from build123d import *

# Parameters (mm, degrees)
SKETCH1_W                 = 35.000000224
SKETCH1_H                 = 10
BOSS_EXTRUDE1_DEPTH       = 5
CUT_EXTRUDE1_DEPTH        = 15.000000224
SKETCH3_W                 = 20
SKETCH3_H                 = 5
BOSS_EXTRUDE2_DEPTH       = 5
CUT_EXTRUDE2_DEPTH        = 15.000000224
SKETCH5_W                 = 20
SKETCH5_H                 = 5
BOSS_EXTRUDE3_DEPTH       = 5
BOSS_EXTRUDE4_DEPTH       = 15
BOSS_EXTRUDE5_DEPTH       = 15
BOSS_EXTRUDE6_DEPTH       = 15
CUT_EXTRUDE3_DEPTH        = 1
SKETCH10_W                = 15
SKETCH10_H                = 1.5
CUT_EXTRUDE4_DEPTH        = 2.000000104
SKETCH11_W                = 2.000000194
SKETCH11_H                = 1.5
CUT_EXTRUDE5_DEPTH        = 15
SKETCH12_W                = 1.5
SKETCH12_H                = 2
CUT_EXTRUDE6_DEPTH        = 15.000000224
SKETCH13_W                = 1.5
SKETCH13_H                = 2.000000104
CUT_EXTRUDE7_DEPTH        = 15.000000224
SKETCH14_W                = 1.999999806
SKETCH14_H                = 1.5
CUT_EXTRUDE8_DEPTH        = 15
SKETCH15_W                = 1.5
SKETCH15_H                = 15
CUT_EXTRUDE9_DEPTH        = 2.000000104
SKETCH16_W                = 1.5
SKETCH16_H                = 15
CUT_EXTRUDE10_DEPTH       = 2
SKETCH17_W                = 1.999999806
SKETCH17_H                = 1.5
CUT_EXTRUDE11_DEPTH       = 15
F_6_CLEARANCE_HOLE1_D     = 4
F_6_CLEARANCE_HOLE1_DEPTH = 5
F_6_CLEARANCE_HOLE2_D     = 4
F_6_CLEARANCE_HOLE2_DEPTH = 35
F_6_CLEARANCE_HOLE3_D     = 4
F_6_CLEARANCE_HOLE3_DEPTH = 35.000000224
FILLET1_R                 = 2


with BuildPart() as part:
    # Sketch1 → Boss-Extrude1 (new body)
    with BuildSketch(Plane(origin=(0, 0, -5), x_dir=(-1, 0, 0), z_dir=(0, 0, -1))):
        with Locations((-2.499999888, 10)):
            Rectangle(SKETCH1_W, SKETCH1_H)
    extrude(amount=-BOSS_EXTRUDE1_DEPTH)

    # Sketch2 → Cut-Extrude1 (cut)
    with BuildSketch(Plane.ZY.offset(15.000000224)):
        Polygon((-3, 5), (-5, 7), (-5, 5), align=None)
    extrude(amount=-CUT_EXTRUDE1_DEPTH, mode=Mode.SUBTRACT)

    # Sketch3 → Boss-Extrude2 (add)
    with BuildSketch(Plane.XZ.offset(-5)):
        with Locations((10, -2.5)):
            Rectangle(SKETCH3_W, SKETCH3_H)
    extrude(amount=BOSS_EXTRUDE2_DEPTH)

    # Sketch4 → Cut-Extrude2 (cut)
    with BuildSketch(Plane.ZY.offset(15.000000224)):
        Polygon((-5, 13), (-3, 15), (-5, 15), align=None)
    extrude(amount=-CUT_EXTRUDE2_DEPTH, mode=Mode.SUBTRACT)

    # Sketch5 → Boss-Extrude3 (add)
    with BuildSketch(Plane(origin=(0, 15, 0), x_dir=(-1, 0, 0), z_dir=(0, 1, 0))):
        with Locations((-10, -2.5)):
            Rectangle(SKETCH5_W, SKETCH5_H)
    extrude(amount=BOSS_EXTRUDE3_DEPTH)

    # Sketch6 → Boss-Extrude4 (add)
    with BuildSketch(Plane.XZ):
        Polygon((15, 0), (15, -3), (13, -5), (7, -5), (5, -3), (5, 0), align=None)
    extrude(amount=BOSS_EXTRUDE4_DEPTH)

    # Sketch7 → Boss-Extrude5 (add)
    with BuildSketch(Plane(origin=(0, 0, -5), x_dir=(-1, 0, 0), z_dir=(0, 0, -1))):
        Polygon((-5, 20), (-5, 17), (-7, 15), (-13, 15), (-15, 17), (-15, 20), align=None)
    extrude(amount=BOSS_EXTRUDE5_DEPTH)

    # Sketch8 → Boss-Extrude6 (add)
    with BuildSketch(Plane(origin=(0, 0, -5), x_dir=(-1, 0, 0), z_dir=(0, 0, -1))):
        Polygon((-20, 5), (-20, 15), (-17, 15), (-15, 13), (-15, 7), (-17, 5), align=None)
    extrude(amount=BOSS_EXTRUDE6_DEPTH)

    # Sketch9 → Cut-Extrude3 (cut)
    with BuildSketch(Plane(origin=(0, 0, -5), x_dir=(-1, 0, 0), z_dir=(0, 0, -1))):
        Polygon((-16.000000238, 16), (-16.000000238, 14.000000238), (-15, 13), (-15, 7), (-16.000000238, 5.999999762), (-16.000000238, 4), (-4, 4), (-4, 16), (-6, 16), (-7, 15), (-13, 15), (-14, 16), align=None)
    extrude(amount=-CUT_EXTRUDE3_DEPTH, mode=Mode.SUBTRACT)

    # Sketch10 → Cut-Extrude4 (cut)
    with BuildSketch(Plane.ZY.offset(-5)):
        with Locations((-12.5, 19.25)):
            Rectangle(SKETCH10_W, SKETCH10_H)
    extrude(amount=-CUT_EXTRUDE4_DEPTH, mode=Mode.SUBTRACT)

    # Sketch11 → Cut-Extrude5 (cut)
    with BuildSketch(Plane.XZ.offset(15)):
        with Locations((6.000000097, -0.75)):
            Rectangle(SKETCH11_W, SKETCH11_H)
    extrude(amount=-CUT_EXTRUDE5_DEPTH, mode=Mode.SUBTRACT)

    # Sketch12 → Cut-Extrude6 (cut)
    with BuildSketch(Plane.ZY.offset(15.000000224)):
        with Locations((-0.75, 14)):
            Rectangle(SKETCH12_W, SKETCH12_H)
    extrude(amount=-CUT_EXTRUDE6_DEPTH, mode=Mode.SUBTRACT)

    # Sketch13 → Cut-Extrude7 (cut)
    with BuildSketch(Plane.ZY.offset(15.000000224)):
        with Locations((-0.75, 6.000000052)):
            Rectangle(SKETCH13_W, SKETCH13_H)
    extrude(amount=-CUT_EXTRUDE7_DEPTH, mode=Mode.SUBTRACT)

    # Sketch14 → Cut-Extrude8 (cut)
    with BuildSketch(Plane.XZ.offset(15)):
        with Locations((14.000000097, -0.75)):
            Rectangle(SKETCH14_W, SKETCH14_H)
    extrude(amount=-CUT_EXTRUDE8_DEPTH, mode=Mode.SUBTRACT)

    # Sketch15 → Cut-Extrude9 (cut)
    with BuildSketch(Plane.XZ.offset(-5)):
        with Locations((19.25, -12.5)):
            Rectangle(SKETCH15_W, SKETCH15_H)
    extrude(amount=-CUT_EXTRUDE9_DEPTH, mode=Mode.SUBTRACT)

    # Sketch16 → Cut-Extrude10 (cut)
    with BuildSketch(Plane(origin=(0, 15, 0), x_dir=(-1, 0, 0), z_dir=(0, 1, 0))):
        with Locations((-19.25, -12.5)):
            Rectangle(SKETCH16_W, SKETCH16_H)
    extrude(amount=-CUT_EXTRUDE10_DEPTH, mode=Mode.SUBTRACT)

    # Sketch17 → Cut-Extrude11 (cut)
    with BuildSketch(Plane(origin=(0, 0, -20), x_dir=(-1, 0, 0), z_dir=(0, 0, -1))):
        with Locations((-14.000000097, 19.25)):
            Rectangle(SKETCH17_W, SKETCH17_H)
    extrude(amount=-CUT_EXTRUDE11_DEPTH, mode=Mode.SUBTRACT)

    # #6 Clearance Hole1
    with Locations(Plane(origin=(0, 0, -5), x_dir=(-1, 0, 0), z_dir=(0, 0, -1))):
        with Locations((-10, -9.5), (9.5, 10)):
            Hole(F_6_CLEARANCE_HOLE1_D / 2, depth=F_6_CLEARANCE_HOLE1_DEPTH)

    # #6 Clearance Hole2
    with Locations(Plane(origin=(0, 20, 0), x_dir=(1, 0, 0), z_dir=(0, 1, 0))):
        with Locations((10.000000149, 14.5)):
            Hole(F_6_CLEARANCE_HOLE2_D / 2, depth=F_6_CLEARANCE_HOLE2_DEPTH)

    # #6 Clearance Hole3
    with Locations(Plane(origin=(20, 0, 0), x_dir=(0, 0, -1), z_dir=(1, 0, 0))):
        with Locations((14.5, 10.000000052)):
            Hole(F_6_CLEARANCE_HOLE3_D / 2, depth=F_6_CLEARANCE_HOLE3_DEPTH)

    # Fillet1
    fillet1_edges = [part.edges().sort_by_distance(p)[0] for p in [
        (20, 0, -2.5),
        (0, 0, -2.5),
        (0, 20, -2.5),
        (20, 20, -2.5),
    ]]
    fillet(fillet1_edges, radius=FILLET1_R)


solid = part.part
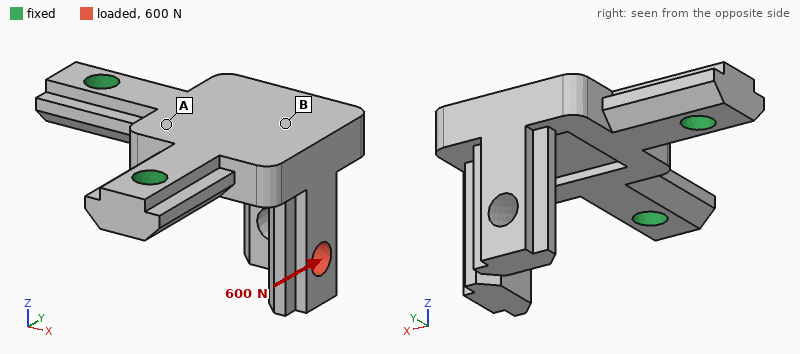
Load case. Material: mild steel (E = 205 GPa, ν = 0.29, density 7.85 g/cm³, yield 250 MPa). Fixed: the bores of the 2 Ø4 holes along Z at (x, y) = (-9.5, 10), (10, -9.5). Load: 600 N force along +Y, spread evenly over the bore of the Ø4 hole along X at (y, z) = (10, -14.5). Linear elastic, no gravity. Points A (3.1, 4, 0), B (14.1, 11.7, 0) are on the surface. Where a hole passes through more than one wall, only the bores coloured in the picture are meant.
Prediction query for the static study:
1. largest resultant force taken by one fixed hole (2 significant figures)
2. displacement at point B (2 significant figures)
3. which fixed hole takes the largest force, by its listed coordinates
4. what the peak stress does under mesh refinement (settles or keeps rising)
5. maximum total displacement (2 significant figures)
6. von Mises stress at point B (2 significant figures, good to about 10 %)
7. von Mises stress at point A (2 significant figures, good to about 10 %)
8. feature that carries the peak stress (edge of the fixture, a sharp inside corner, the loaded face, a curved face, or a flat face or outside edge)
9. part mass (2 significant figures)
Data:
710 N
33 µm
(10, -9.5)
keeps rising
96 µm
69 MPa
25 MPa
a sharp inside corner
31 g
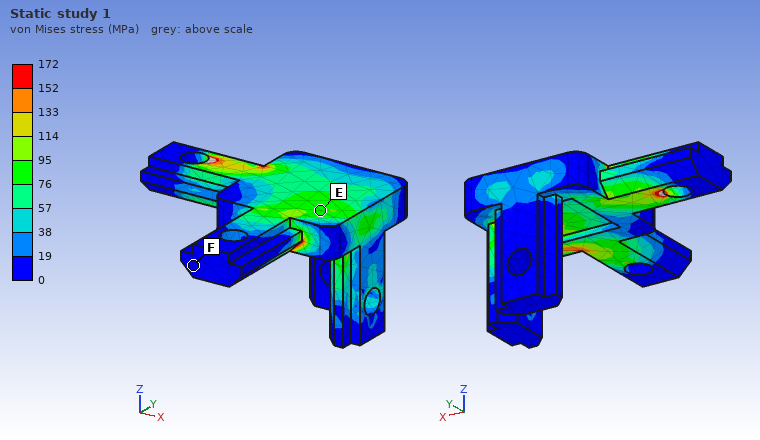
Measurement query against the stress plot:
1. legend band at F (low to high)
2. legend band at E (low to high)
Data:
0 to 19 MPa
76 to 95 MPa
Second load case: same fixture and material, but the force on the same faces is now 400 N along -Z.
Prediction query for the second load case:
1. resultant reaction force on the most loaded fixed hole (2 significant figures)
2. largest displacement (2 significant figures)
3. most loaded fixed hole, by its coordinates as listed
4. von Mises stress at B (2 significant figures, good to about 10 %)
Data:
290 N
70 µm
(10, -9.5)
25 MPa
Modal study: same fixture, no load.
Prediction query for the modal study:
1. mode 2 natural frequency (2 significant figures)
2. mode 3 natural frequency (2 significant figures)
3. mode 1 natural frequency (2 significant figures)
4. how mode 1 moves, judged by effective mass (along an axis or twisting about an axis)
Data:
7500 Hz
10 kHz
3500 Hz
along Z
